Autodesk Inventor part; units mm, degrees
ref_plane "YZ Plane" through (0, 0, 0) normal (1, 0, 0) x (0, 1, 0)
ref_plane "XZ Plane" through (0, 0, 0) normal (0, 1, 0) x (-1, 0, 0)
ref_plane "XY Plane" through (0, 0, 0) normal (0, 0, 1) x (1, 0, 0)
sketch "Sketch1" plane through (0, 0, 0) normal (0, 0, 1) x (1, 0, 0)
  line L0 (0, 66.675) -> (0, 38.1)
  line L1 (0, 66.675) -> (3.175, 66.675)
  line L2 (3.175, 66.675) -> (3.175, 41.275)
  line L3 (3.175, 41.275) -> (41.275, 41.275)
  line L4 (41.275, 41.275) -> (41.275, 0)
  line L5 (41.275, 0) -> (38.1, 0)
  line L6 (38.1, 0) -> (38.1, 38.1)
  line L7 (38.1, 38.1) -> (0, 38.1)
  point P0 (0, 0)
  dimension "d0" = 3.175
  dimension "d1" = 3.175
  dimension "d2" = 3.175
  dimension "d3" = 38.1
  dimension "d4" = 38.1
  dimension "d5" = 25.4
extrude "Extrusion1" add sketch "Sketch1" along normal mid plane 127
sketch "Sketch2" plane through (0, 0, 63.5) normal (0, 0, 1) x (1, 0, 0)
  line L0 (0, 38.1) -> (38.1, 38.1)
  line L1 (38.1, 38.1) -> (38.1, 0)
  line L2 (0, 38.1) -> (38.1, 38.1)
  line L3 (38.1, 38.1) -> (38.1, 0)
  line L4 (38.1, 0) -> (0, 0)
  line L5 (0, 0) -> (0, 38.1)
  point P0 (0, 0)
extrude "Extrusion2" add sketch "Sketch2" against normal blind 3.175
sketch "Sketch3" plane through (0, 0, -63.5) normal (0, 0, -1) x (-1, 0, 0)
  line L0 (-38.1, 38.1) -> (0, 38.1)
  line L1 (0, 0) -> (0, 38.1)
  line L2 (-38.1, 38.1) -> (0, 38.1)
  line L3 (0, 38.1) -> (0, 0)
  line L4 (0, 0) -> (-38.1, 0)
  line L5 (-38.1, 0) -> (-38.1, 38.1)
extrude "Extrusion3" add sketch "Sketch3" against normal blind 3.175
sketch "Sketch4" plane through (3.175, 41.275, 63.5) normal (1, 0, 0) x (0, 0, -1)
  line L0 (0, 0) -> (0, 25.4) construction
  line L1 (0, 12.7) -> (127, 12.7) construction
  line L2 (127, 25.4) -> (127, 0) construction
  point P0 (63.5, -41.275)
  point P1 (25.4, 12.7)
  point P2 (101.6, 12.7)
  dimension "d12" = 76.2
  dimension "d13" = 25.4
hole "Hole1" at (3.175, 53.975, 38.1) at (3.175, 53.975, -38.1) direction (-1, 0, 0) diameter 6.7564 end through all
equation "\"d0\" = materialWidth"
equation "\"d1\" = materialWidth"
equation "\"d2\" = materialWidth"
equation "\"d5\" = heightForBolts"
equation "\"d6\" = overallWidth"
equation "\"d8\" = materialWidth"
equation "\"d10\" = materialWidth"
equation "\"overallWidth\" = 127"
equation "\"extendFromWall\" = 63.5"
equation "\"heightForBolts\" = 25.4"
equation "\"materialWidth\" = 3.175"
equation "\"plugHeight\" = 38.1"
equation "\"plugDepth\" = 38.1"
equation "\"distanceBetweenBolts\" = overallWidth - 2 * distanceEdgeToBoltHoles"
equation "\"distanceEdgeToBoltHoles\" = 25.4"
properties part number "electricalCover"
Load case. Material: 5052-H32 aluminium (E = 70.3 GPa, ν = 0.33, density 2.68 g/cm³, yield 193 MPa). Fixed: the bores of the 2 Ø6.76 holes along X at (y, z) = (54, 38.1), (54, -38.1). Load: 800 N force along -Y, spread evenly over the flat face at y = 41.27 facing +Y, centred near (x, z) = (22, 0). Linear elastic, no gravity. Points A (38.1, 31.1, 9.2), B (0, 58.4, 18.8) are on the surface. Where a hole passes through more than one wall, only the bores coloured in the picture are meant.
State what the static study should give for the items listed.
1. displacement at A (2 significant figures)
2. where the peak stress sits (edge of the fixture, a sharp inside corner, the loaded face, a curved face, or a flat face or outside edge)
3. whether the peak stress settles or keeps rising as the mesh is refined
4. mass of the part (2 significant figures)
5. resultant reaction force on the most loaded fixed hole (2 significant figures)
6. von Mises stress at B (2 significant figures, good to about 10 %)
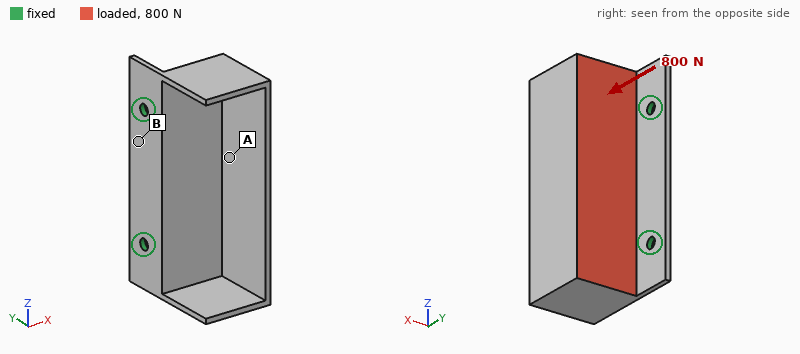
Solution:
0.60 mm
edge of the fixture
keeps rising
140 g
400 N
30 MPa
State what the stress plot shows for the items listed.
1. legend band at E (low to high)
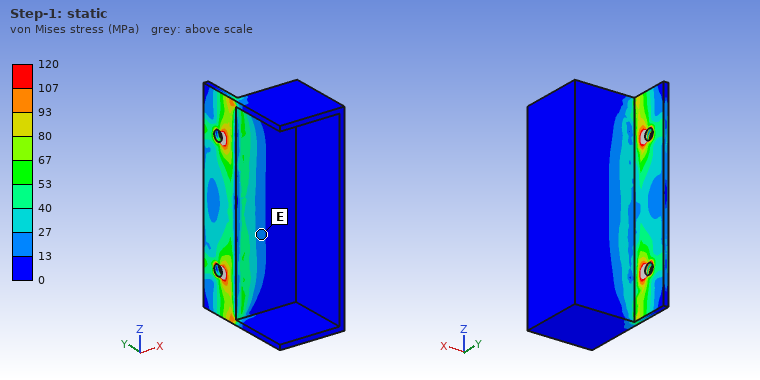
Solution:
13 to 27 MPa
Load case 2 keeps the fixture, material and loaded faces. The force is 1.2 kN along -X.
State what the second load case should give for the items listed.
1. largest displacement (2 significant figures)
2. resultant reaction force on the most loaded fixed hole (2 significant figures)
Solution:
0.30 mm
600 N
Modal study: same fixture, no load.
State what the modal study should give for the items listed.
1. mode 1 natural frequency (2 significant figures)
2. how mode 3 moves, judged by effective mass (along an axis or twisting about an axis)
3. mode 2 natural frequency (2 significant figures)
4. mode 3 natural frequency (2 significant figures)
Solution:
410 Hz
along Z
660 Hz
1900 Hz
